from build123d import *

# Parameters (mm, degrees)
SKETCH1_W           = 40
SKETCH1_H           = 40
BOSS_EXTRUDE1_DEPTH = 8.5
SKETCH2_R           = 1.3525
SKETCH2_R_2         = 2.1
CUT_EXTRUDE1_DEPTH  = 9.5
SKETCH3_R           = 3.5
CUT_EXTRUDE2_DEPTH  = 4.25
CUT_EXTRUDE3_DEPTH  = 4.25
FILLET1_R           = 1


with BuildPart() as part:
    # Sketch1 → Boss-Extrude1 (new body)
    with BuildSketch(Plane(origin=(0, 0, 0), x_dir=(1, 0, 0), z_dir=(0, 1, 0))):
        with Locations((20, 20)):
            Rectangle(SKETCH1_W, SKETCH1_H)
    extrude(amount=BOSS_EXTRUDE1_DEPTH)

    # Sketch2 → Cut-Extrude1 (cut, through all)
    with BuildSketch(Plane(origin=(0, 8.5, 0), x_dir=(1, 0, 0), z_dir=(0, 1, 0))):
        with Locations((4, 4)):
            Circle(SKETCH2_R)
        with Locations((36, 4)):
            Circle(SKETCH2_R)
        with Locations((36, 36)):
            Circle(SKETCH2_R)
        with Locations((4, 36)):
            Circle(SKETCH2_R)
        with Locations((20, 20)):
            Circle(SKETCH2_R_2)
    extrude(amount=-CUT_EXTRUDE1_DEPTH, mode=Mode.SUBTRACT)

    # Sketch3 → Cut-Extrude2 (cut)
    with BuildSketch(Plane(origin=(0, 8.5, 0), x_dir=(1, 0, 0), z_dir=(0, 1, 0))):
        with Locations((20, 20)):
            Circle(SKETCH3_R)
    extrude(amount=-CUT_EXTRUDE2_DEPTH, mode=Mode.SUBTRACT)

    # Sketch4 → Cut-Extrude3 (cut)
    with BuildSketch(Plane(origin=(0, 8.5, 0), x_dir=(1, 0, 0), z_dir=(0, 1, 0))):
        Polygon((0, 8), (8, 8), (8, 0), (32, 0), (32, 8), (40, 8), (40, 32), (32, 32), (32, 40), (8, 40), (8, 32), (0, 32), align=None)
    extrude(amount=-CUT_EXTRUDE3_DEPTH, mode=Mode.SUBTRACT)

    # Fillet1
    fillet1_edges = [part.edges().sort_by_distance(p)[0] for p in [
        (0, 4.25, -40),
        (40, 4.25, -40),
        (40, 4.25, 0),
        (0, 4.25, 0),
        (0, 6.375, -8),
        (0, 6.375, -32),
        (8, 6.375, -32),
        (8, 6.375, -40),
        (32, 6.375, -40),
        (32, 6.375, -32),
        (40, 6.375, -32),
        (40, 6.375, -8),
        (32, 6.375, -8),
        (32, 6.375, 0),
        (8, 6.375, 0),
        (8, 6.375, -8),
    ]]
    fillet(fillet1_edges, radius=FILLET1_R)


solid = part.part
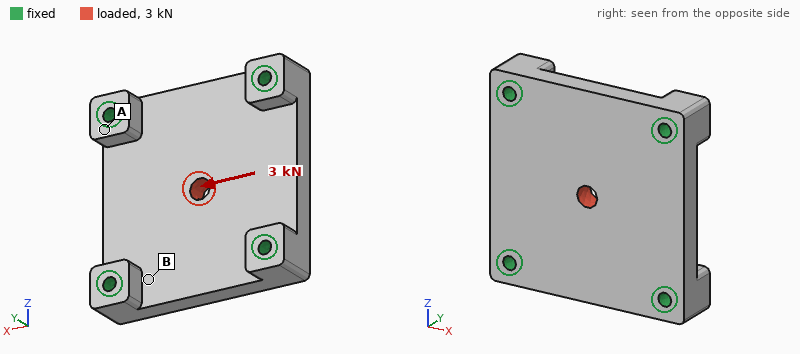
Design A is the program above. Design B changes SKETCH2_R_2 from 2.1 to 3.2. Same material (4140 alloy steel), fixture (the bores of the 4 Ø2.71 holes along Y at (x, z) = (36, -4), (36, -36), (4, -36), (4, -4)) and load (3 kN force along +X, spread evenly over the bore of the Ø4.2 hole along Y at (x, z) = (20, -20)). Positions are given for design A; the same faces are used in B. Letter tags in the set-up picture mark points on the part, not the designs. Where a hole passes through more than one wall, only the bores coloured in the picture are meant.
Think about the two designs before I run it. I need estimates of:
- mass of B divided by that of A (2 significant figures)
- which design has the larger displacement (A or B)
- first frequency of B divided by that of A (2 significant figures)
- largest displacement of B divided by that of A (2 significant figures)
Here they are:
0.99
A
1.0
0.88
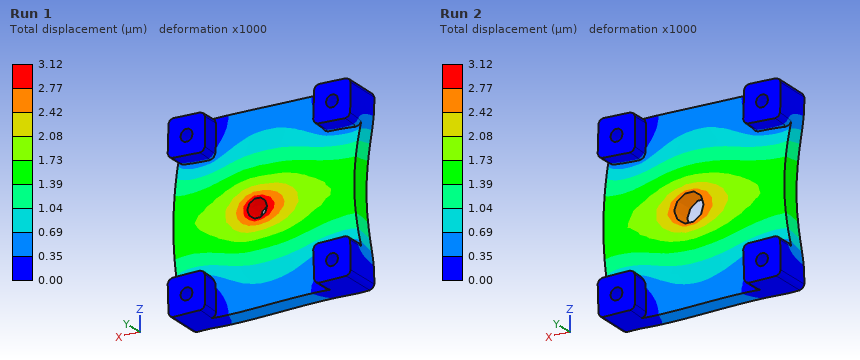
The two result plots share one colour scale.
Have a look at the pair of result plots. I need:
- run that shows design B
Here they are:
Run 2
